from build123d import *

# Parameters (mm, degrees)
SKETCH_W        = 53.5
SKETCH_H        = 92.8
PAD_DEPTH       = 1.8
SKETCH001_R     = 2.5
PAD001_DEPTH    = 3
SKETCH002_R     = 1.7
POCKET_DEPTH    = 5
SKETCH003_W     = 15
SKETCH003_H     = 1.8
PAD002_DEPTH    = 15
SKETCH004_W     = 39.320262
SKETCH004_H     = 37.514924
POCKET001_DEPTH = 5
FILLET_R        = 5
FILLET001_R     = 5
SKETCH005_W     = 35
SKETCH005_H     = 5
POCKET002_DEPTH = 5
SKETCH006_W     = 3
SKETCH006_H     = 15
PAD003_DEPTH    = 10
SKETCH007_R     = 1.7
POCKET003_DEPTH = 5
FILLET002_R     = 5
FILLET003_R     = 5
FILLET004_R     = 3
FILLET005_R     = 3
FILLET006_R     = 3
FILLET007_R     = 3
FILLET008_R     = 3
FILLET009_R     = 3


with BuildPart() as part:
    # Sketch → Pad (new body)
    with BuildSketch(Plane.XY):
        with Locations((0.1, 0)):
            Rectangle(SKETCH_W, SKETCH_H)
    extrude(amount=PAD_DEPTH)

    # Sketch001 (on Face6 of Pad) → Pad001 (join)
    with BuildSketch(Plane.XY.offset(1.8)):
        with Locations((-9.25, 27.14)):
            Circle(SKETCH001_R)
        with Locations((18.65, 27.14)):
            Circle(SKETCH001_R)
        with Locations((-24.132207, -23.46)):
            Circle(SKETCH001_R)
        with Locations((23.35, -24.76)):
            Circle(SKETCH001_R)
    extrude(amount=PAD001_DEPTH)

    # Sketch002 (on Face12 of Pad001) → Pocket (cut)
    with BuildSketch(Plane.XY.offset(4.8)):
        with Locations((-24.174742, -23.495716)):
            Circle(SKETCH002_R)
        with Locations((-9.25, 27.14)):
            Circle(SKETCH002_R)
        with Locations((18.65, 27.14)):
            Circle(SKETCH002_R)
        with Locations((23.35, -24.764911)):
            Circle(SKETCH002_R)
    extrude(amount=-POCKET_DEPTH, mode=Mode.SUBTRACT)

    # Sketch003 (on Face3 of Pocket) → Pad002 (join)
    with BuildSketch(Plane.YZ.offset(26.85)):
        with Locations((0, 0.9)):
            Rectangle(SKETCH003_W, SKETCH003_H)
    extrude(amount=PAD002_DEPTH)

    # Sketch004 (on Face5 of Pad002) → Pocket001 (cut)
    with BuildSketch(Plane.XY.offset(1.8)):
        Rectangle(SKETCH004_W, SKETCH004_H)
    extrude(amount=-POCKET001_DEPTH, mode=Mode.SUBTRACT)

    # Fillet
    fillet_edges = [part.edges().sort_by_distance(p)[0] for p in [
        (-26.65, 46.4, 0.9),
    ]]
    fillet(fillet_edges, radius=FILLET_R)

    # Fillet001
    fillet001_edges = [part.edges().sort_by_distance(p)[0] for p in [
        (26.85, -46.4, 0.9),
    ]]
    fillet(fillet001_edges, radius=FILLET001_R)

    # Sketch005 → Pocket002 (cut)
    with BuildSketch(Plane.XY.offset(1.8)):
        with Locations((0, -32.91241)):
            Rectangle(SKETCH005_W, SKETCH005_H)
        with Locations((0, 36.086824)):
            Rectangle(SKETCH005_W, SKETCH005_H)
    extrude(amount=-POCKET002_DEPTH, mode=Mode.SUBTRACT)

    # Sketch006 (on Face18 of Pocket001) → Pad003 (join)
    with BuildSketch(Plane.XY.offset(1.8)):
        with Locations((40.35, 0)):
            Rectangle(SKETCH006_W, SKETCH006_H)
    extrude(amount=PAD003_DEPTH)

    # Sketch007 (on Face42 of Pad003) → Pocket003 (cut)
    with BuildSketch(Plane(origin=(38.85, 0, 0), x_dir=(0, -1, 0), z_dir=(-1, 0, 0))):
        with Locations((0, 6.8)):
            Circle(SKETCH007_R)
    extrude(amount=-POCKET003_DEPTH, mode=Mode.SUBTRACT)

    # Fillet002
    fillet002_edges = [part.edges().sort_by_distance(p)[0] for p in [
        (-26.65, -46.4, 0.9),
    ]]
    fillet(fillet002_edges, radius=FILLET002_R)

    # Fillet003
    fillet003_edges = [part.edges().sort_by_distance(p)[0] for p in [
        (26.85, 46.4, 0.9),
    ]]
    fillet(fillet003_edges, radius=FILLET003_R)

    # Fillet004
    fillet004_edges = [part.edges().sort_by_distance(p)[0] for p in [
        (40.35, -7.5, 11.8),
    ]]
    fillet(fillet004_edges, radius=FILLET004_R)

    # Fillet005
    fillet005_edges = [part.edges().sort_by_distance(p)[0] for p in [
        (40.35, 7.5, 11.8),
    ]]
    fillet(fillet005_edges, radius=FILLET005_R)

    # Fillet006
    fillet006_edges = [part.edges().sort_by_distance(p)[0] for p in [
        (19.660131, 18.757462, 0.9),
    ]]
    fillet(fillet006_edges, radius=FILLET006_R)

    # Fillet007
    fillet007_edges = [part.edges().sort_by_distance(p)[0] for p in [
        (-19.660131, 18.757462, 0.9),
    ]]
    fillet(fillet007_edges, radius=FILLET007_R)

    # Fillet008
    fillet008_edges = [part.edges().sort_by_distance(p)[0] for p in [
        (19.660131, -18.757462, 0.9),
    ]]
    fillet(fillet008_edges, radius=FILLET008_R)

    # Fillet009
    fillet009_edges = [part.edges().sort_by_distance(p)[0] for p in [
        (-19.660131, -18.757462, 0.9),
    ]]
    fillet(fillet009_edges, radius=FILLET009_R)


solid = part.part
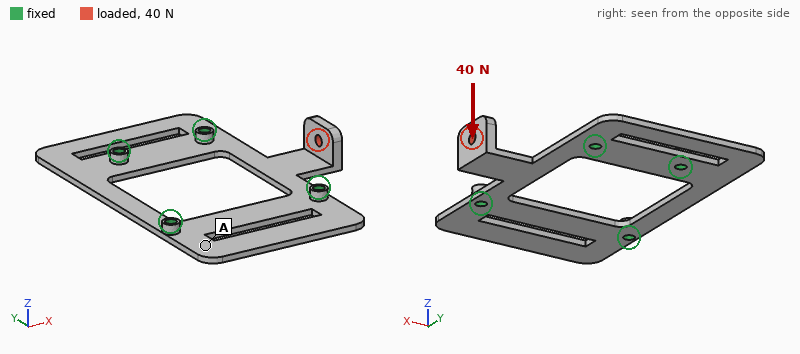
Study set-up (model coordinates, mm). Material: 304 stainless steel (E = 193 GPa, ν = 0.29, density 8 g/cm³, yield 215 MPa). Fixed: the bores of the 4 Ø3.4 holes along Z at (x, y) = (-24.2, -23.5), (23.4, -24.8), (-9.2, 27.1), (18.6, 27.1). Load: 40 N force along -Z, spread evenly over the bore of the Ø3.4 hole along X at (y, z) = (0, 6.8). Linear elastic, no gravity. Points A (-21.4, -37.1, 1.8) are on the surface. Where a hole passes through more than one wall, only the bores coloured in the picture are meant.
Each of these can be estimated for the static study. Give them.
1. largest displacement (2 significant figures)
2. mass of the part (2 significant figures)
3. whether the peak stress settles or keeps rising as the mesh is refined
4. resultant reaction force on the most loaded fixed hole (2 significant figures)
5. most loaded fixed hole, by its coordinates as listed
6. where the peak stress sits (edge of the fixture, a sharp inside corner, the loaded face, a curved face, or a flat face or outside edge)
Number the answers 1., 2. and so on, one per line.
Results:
1. 0.22 mm
2. 52 g
3. keeps rising
4. 24 N
5. (23.4, -24.8)
6. a sharp inside corner
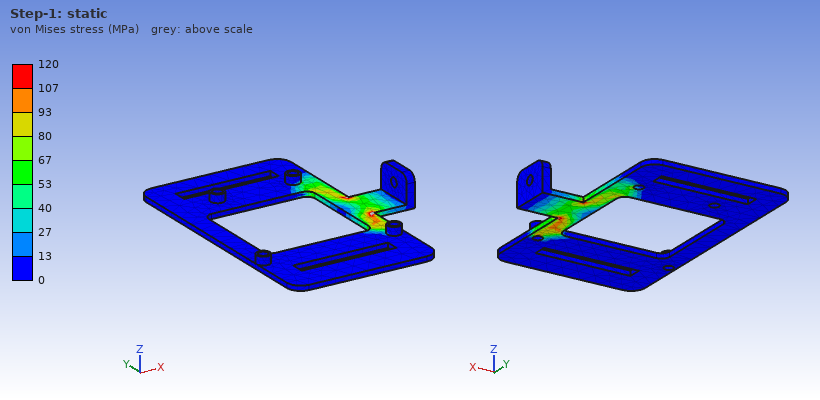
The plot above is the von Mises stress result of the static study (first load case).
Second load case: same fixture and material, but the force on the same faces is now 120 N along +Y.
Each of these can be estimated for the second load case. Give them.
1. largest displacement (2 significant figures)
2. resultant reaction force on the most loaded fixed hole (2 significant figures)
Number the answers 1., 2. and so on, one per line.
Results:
1. 71 µm
2. 78 N
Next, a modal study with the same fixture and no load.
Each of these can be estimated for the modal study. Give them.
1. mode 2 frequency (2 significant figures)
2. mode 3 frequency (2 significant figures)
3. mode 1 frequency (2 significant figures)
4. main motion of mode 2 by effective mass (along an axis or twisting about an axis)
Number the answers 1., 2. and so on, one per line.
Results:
1. 1800 Hz
2. 2200 Hz
3. 1000 Hz
4. along Z
